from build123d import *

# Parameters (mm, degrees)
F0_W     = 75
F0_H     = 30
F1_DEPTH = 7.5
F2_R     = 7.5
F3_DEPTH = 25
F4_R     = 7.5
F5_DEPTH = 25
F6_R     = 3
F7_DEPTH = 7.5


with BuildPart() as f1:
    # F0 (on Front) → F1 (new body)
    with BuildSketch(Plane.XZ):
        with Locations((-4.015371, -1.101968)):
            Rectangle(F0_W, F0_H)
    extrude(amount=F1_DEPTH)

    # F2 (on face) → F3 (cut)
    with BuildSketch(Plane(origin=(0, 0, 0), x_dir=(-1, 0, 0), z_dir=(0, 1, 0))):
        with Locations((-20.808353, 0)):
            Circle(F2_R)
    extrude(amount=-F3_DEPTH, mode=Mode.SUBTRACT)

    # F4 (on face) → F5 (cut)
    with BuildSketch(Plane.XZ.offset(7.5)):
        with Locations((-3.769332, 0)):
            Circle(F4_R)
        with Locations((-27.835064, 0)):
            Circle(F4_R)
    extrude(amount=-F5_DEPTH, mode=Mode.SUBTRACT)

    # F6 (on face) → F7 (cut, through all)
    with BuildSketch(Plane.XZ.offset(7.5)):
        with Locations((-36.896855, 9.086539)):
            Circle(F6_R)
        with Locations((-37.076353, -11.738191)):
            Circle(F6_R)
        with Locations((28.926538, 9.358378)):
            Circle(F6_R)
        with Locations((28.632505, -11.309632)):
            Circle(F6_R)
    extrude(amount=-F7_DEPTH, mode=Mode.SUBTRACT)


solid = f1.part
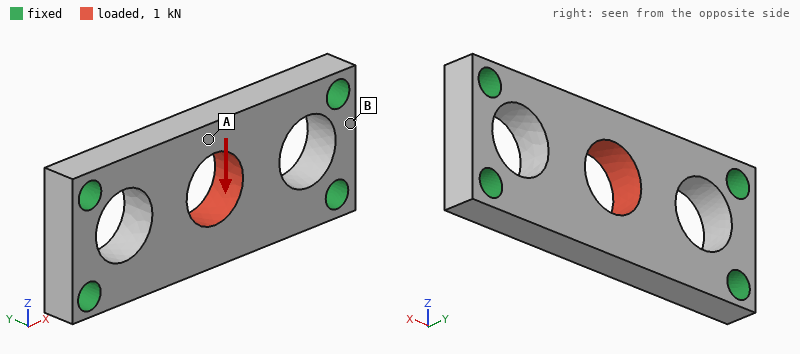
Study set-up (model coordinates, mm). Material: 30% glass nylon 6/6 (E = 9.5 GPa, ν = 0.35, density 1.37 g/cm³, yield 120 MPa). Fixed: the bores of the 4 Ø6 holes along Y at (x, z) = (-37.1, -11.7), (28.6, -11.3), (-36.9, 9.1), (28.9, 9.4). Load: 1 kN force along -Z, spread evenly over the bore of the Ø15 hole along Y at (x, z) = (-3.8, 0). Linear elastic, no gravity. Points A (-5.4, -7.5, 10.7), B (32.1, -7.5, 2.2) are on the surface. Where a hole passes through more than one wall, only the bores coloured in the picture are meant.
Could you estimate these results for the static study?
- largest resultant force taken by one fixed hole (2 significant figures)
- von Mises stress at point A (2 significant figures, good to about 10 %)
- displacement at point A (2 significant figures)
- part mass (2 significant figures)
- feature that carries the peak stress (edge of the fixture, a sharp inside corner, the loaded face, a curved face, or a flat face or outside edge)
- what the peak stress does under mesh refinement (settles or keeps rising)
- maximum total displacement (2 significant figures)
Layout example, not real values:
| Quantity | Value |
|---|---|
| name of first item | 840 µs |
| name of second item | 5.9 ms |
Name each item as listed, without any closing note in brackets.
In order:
| Quantity | Value |
|---|---|
| largest resultant force taken by one fixed hole | 380 N |
| von Mises stress at point A | 5.3 MPa |
| displacement at point A | 61 µm |
| part mass | 17 g |
| feature that carries the peak stress | edge of the fixture |
| what the peak stress does under mesh refinement | keeps rising |
| maximum total displacement | 62 µm |
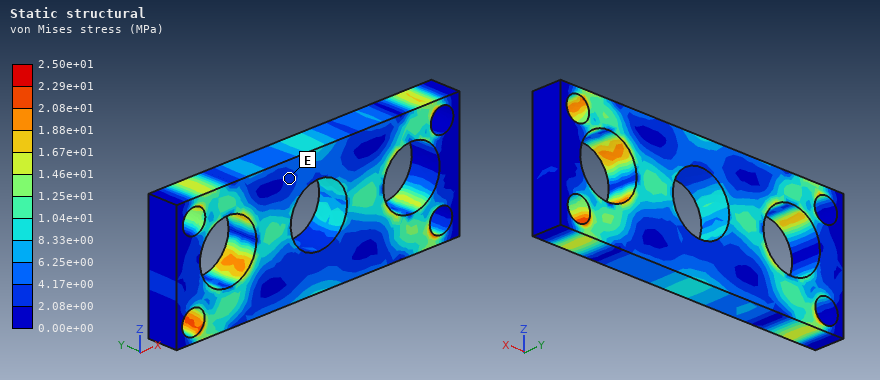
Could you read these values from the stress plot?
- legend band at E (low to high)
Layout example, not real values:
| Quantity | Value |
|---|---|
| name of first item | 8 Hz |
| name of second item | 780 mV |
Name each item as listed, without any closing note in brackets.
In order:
| Quantity | Value |
|---|---|
| legend band at E | 2.08e+00 to 4.17e+00 MPa |
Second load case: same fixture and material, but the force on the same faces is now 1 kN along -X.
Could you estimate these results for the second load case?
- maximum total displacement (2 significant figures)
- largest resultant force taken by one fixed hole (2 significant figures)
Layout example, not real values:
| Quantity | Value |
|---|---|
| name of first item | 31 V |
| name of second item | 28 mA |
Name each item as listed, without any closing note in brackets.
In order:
| Quantity | Value |
|---|---|
| maximum total displacement | 13 µm |
| largest resultant force taken by one fixed hole | 270 N |
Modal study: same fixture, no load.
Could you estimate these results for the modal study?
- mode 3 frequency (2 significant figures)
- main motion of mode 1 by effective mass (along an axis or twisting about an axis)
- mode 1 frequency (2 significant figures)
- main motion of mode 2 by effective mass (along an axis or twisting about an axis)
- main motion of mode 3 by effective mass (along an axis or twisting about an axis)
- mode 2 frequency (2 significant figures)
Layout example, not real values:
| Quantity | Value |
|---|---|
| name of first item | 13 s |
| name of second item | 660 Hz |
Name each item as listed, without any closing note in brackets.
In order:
| Quantity | Value |
|---|---|
| mode 3 frequency | 7200 Hz |
| main motion of mode 1 by effective mass | along Y |
| mode 1 frequency | 4300 Hz |
| main motion of mode 2 by effective mass | twisting about X |
| main motion of mode 3 by effective mass | along Z |
| mode 2 frequency | 6400 Hz |
